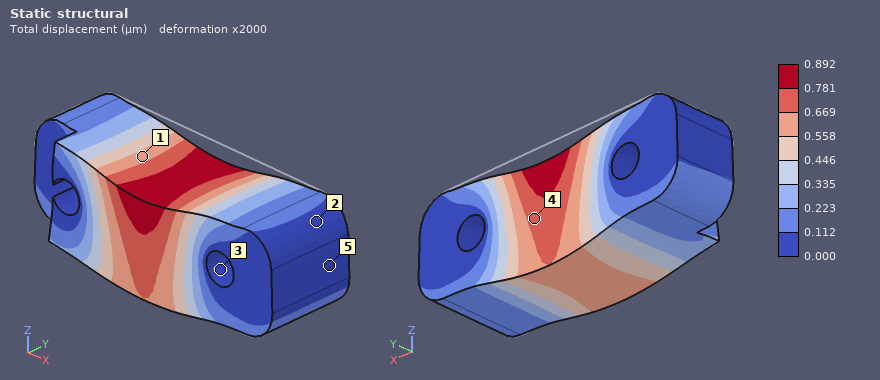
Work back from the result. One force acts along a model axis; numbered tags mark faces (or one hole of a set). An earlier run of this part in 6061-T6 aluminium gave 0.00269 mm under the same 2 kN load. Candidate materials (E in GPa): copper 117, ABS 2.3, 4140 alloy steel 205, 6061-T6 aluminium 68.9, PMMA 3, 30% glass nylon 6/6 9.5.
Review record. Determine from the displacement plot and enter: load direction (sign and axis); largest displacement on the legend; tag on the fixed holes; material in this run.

-Z
0.892 µm
3
4140 alloy steel
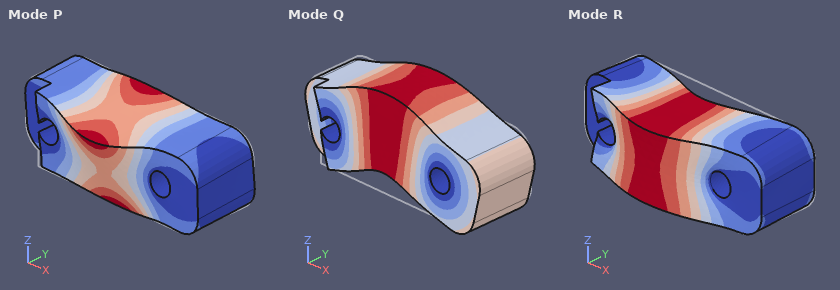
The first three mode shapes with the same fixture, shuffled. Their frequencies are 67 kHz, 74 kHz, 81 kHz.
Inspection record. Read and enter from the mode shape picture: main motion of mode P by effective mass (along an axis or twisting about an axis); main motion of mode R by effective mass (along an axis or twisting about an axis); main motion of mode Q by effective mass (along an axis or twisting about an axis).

twisting about X
along Y
along Z
